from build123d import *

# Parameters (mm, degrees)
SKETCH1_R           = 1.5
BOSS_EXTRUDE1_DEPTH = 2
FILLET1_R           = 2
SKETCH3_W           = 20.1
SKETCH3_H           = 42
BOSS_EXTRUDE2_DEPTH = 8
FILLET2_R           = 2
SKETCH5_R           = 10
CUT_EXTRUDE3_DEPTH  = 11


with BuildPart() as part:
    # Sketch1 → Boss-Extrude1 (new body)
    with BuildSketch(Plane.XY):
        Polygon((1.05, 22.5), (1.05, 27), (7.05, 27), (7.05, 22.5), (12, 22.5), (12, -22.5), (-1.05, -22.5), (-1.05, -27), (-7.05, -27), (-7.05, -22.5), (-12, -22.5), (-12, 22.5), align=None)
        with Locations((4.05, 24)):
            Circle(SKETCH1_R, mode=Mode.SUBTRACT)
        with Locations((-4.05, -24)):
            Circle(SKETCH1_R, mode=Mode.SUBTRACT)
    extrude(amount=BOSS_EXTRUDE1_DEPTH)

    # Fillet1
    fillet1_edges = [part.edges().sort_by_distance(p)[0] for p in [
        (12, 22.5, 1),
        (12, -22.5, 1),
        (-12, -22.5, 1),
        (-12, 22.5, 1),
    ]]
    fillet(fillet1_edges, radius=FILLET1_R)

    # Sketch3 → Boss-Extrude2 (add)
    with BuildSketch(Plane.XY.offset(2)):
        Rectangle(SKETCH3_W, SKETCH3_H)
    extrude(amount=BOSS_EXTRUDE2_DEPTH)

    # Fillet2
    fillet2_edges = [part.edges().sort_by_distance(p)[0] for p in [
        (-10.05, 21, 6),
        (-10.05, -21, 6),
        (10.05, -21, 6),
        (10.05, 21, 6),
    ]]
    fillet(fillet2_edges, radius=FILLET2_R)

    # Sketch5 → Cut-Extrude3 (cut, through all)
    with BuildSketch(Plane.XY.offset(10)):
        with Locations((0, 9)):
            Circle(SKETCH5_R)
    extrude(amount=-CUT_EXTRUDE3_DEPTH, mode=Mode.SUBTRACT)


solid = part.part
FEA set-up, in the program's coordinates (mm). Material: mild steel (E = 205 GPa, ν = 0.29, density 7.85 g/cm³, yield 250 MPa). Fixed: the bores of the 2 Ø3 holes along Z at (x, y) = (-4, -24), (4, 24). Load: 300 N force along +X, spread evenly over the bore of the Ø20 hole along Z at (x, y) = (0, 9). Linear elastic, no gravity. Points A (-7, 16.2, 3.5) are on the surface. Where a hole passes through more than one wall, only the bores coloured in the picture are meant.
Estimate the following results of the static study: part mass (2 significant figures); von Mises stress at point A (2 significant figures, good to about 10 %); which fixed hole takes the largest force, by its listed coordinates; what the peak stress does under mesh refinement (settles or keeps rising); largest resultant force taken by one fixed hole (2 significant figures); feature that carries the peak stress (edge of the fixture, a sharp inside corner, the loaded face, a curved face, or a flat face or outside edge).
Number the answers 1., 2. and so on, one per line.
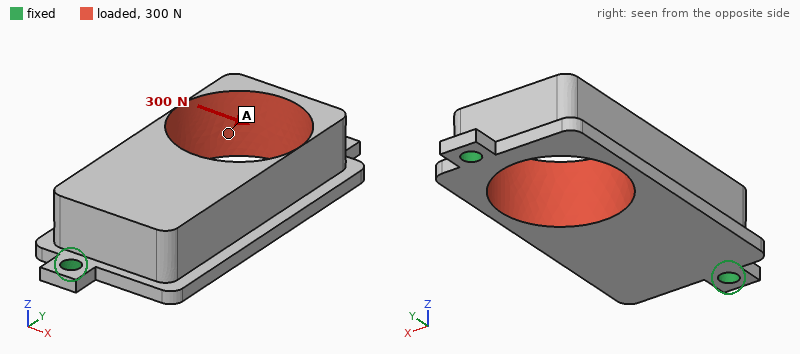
1. 46 g
2. 11 MPa
3. (4, 24)
4. keeps rising
5. 200 N
6. edge of the fixture
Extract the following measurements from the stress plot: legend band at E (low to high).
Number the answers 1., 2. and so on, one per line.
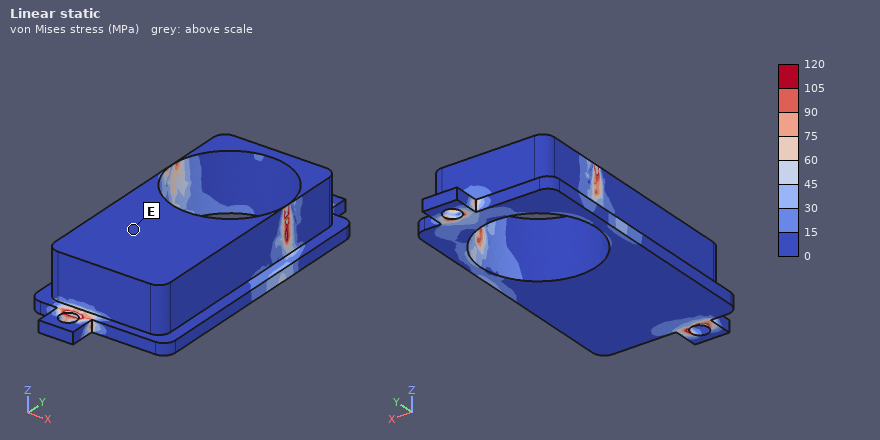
1. 0 to 15 MPa
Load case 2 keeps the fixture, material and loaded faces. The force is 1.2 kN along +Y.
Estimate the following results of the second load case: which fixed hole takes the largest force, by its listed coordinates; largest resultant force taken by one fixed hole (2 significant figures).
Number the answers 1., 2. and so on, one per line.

1. (-4, -24)
2. 750 N
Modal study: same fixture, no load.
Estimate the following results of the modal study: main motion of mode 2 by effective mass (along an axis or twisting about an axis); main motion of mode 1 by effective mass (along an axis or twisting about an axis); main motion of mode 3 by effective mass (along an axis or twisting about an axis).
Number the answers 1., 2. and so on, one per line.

1. along Z
2. along X
3. along X
